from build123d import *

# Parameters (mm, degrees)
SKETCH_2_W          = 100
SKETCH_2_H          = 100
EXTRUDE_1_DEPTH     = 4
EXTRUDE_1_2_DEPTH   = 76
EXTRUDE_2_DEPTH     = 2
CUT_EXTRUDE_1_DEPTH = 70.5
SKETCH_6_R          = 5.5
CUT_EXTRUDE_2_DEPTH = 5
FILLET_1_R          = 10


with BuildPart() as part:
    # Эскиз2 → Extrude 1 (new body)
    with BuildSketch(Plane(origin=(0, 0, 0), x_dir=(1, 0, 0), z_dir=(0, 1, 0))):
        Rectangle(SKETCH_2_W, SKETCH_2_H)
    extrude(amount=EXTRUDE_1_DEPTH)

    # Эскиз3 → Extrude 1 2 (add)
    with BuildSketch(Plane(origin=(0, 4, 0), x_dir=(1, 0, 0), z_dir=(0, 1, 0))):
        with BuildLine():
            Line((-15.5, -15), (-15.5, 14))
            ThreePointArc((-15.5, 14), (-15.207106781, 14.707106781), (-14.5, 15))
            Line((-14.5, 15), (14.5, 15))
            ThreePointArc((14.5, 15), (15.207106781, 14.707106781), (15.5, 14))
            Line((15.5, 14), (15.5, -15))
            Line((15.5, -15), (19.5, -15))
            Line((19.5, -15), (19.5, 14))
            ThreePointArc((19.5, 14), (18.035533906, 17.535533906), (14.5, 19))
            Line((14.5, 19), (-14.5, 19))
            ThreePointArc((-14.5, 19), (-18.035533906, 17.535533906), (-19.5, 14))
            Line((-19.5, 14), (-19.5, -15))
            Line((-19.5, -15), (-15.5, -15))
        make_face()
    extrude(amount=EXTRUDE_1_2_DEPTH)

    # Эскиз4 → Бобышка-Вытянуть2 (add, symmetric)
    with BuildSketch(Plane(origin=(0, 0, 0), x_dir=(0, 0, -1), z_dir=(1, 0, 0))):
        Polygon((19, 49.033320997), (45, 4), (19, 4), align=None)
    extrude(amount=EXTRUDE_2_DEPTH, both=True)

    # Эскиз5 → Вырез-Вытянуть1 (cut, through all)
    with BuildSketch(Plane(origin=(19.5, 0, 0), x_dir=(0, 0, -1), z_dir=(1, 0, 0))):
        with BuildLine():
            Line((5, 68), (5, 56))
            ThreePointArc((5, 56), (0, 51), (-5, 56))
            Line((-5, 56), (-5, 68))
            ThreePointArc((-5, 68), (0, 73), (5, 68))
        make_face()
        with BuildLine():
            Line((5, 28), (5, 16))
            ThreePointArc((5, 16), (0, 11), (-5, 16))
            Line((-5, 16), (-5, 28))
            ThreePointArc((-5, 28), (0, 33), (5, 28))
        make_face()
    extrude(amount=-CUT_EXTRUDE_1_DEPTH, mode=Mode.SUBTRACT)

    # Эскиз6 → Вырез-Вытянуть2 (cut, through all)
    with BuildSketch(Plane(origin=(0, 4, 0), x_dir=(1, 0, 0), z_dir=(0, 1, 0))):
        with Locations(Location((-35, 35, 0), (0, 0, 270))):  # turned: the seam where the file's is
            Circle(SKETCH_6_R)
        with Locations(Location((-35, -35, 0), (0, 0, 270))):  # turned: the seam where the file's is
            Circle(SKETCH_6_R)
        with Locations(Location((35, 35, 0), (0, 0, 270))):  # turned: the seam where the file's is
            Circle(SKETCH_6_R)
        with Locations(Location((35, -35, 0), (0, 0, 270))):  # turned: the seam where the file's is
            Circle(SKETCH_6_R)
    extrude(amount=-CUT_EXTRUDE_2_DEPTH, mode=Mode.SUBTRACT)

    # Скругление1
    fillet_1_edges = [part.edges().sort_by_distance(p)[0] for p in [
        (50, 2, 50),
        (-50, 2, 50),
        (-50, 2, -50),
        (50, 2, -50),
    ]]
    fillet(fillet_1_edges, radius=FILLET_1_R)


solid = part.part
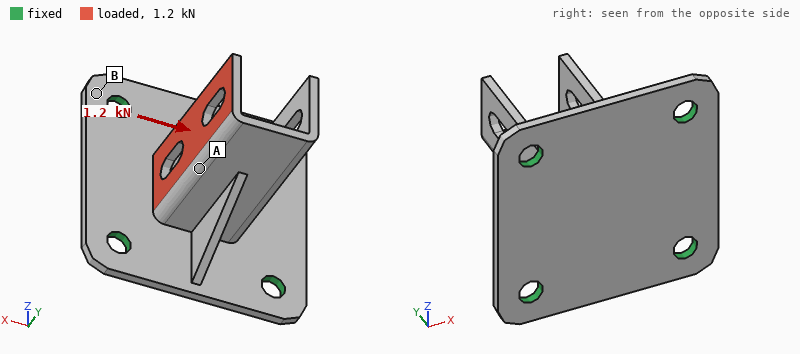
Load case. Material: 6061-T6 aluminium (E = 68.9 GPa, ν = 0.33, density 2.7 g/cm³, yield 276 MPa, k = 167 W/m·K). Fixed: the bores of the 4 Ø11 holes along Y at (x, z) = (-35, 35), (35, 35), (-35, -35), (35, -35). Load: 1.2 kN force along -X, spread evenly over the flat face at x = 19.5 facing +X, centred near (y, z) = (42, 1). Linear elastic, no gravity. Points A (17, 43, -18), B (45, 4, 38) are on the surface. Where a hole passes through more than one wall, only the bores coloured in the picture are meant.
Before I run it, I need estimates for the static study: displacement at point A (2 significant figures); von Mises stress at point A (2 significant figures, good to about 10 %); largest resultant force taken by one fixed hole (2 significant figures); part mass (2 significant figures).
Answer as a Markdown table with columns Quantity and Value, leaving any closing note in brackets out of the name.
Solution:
| Quantity | Value |
|---|---|
| displacement at point A | 0.17 mm |
| von Mises stress at point A | 37 MPa |
| largest resultant force taken by one fixed hole | 820 N |
| part mass | 180 g |
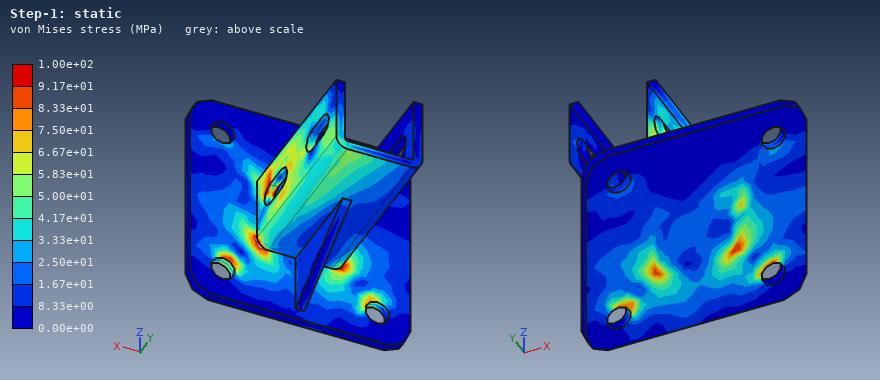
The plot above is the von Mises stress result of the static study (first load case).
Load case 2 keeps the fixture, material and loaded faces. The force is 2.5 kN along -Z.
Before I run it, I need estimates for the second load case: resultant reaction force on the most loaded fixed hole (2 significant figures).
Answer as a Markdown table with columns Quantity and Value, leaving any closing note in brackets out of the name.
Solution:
| Quantity | Value |
|---|---|
| resultant reaction force on the most loaded fixed hole | 1.5 kN |
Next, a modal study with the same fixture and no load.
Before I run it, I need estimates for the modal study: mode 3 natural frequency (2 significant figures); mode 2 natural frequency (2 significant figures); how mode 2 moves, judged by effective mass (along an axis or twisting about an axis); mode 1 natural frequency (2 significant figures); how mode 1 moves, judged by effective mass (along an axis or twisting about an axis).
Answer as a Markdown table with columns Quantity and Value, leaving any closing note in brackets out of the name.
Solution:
| Quantity | Value |
|---|---|
| mode 3 natural frequency | 2400 Hz |
| mode 2 natural frequency | 1800 Hz |
| how mode 2 moves, judged by effective mass | along Z |
| mode 1 natural frequency | 1300 Hz |
| how mode 1 moves, judged by effective mass | along X |
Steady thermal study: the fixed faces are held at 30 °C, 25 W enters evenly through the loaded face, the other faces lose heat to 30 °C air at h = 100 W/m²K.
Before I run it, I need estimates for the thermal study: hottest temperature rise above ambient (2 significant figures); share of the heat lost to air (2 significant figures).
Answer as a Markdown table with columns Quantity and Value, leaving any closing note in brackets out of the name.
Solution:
| Quantity | Value |
|---|---|
| hottest temperature rise above ambient | 21 K |
| share of the heat lost to air | 56 % |
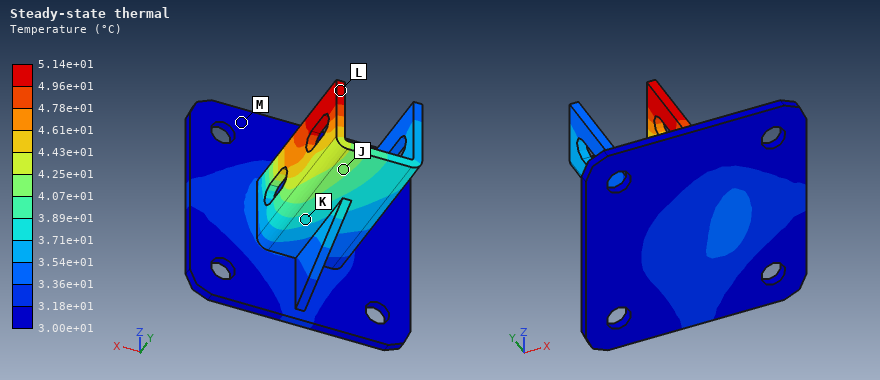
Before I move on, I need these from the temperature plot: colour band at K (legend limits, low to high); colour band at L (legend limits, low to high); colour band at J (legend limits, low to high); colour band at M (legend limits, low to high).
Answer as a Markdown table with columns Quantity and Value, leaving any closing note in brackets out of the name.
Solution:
| Quantity | Value |
|---|---|
| colour band at K | 3.71e+01 to 3.89e+01 °C |
| colour band at L | 4.96e+01 to 5.14e+01 °C |
| colour band at J | 4.07e+01 to 4.25e+01 °C |
| colour band at M | 3.00e+01 to 3.18e+01 °C |
